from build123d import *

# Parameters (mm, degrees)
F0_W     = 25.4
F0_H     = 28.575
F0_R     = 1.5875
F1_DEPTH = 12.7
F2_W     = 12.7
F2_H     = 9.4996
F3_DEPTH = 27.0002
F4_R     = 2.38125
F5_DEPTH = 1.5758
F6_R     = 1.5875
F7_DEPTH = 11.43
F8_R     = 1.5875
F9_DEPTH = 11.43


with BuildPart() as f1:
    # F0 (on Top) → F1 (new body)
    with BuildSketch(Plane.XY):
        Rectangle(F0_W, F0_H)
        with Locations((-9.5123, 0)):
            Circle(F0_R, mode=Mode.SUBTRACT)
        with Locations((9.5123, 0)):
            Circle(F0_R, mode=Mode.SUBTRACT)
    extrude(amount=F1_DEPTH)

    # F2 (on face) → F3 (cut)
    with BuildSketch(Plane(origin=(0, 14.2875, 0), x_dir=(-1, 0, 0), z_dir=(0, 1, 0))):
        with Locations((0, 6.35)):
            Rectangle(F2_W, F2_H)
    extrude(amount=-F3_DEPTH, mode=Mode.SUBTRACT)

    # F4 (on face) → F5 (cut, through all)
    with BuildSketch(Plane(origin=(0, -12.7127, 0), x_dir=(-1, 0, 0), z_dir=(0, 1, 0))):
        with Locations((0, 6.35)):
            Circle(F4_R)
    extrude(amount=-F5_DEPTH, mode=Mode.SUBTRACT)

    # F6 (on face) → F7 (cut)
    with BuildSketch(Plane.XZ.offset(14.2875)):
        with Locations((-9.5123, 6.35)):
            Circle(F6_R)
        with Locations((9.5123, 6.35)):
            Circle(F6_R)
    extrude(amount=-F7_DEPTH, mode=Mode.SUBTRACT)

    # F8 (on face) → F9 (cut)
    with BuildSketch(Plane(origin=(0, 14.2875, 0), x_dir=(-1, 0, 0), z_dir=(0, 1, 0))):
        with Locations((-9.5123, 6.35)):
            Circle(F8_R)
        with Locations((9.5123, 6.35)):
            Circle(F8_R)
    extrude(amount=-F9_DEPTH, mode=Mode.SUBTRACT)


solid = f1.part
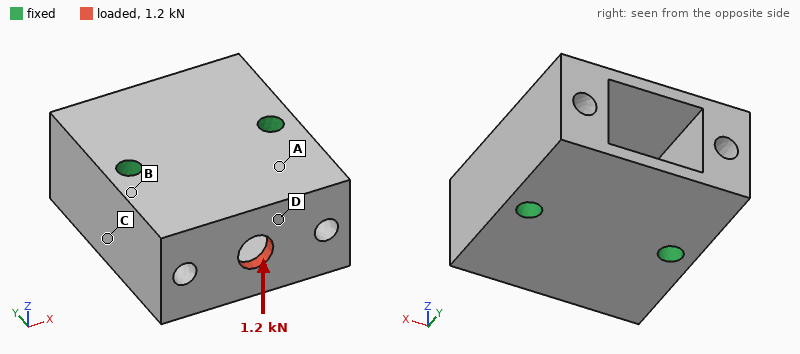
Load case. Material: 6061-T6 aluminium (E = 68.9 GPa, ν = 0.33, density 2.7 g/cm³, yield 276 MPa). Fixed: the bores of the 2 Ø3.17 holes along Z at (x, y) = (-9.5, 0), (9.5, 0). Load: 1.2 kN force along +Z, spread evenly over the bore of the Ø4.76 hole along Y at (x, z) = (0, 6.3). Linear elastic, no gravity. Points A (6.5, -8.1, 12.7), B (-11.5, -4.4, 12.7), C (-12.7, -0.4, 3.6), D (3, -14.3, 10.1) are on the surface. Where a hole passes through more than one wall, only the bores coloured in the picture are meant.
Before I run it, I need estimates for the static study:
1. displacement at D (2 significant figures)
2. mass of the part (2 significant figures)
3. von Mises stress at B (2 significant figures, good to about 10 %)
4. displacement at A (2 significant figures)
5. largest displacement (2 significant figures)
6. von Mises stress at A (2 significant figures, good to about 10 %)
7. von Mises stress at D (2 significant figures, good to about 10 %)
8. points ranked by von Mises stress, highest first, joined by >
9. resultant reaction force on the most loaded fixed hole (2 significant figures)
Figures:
19 µm
14 g
31 MPa
7.1 µm
23 µm
19 MPa
55 MPa
D > B > A > C
600 N
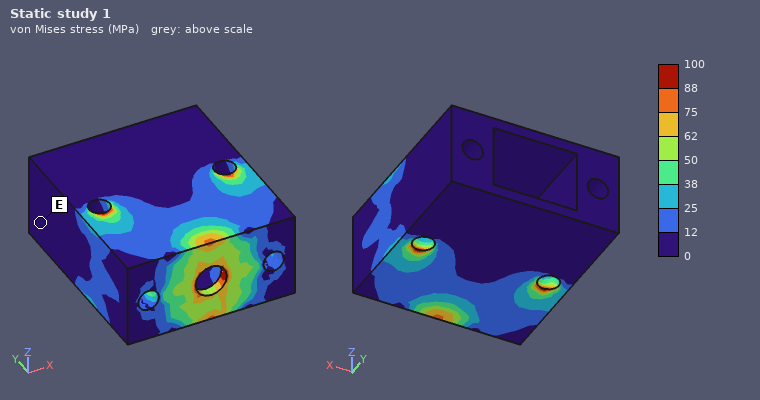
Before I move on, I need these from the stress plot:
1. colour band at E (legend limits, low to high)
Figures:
0 to 12 MPa
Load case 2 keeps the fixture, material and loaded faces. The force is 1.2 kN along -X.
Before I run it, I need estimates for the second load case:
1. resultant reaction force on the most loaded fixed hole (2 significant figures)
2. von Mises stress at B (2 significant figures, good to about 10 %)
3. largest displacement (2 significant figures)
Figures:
890 N
14 MPa
11 µm
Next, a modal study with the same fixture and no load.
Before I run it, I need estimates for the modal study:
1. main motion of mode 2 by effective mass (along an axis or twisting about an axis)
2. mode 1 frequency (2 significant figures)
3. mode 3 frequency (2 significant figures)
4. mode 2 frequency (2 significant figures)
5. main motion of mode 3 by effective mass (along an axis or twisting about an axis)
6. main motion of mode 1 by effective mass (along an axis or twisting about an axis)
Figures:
along Z
29 kHz
36 kHz
31 kHz
along X
twisting about X
